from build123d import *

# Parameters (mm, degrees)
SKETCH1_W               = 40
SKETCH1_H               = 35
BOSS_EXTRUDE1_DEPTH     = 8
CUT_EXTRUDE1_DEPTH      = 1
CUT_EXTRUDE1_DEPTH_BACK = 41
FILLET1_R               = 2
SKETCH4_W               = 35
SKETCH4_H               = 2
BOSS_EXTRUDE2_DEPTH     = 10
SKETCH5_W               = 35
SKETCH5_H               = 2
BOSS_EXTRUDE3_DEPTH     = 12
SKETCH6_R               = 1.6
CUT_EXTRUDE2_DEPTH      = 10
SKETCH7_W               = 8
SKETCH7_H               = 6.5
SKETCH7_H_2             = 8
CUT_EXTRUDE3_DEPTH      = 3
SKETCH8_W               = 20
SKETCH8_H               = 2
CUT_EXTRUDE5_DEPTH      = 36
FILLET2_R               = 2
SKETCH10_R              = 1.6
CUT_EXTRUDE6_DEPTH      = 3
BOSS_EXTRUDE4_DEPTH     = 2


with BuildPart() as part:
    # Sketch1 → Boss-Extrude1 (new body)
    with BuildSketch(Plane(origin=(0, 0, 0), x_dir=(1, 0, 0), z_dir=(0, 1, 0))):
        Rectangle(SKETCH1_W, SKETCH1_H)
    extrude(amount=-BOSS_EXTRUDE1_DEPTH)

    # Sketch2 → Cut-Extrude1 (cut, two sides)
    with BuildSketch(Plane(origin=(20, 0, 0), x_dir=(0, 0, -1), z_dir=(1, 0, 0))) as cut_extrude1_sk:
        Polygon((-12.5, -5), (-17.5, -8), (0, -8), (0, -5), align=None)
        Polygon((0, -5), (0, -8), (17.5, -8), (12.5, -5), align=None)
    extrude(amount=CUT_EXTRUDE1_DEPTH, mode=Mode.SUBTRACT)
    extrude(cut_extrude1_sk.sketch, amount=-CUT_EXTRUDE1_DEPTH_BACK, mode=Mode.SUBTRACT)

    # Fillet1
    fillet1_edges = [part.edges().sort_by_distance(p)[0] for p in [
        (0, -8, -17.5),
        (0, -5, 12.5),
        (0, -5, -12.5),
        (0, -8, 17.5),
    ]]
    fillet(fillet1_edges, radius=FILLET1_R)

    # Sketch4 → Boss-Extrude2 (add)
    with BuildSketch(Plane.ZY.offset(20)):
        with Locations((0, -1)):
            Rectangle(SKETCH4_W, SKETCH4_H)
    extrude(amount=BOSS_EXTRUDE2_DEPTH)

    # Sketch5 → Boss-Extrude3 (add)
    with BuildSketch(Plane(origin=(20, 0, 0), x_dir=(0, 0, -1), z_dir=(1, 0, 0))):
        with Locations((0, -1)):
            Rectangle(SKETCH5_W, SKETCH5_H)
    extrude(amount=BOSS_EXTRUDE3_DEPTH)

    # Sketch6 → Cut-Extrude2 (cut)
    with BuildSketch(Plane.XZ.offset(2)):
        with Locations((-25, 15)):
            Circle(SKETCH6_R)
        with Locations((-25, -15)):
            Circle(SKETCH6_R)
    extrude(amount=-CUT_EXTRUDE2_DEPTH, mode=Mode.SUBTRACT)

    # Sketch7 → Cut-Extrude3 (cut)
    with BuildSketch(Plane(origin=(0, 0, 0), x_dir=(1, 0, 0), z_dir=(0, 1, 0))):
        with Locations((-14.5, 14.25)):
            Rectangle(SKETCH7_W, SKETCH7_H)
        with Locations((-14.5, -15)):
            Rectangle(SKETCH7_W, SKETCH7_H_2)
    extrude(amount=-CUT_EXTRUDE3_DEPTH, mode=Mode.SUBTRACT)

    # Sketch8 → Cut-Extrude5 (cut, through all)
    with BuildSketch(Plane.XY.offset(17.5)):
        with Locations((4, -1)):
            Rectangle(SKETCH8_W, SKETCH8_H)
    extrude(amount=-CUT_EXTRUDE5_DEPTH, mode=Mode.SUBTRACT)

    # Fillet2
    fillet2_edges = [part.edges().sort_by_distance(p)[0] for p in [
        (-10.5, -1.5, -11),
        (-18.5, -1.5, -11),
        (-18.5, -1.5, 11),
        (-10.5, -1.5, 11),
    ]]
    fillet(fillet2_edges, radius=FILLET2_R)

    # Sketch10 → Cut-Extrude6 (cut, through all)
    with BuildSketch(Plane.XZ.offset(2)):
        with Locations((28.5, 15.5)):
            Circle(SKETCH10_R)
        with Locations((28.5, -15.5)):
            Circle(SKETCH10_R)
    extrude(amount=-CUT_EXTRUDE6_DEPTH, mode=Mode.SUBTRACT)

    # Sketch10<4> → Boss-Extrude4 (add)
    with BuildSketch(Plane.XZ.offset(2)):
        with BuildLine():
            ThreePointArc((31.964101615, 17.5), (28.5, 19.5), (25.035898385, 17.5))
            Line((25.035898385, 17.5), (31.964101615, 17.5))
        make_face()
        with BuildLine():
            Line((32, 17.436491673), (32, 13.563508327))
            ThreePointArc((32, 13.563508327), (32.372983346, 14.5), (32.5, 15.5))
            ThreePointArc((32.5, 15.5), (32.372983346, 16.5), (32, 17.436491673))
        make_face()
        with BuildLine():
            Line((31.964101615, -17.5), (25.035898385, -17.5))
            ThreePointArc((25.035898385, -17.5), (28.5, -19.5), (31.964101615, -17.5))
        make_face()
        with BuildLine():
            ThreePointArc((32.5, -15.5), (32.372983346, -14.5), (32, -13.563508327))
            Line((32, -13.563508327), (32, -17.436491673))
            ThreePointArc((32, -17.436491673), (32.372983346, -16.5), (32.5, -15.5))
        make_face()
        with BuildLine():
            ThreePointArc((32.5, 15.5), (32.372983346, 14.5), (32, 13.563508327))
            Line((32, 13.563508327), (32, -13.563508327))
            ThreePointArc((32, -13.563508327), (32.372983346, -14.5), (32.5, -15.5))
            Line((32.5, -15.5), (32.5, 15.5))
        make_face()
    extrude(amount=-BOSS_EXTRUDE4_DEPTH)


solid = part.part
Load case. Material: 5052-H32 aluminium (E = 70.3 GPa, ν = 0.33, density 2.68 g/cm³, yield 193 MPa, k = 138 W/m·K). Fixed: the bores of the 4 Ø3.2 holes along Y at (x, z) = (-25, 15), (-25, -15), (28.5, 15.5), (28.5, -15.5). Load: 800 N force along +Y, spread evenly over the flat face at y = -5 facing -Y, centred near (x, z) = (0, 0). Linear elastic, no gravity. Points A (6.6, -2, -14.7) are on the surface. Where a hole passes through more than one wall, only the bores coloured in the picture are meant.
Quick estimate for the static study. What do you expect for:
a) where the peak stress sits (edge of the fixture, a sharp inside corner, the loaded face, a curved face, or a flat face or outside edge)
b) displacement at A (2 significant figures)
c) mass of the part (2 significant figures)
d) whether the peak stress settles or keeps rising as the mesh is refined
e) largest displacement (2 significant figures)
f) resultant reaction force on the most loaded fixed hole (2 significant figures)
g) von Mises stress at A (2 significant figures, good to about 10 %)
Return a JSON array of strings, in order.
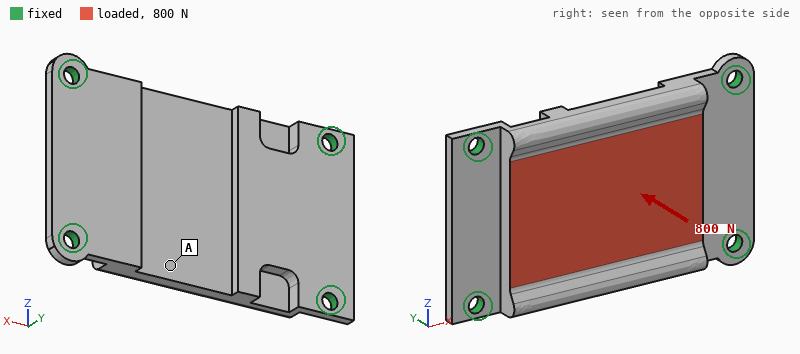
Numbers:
["edge of the fixture", "55 µm", "19 g", "keeps rising", "65 µm", "570 N", "18 MPa"]
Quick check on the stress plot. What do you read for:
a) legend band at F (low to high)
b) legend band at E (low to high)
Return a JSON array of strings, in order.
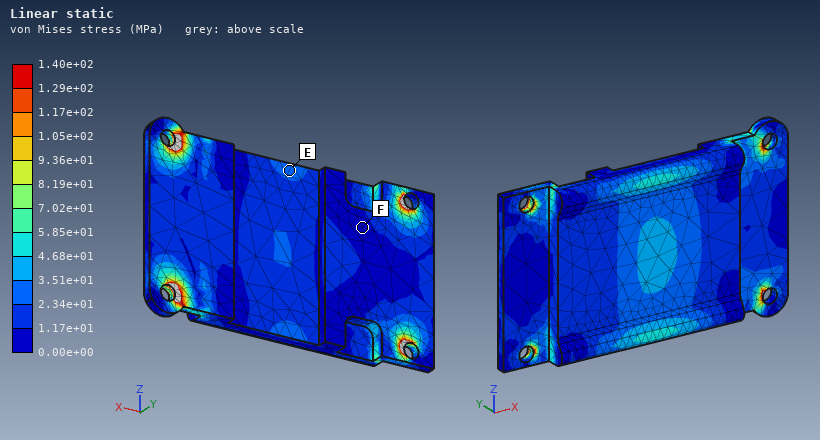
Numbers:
["0.00e+00 to 1.17e+01 MPa", "2.34e+01 to 3.51e+01 MPa"]
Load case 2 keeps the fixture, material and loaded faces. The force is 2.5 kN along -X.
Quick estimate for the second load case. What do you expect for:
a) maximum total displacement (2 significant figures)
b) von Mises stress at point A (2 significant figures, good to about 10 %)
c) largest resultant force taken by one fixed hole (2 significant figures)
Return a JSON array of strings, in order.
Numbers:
["15 µm", "15 MPa", "680 N"]
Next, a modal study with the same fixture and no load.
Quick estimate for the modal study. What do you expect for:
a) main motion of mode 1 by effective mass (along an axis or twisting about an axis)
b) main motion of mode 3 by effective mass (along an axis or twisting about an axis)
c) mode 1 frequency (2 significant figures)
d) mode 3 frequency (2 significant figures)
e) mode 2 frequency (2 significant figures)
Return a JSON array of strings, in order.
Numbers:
["along Y", "twisting about Z", "5300 Hz", "11 kHz", "8300 Hz"]
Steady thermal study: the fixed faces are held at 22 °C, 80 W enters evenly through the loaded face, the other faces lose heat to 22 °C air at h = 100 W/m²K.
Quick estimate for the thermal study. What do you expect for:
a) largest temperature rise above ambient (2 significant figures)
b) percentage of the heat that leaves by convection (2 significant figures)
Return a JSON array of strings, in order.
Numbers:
["62 K", "21 %"]
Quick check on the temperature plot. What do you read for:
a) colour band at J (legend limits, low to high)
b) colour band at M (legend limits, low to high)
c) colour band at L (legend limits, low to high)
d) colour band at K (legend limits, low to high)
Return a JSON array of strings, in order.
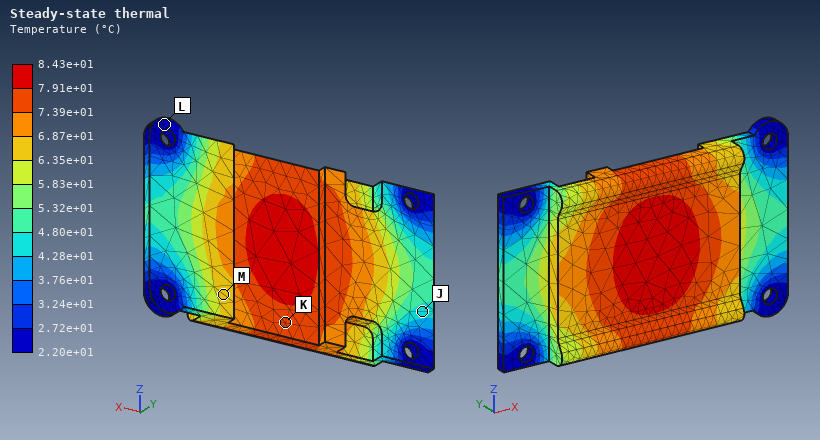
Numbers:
["4.28e+01 to 4.80e+01 °C", "6.35e+01 to 6.87e+01 °C", "2.20e+01 to 2.72e+01 °C", "7.39e+01 to 7.91e+01 °C"]
